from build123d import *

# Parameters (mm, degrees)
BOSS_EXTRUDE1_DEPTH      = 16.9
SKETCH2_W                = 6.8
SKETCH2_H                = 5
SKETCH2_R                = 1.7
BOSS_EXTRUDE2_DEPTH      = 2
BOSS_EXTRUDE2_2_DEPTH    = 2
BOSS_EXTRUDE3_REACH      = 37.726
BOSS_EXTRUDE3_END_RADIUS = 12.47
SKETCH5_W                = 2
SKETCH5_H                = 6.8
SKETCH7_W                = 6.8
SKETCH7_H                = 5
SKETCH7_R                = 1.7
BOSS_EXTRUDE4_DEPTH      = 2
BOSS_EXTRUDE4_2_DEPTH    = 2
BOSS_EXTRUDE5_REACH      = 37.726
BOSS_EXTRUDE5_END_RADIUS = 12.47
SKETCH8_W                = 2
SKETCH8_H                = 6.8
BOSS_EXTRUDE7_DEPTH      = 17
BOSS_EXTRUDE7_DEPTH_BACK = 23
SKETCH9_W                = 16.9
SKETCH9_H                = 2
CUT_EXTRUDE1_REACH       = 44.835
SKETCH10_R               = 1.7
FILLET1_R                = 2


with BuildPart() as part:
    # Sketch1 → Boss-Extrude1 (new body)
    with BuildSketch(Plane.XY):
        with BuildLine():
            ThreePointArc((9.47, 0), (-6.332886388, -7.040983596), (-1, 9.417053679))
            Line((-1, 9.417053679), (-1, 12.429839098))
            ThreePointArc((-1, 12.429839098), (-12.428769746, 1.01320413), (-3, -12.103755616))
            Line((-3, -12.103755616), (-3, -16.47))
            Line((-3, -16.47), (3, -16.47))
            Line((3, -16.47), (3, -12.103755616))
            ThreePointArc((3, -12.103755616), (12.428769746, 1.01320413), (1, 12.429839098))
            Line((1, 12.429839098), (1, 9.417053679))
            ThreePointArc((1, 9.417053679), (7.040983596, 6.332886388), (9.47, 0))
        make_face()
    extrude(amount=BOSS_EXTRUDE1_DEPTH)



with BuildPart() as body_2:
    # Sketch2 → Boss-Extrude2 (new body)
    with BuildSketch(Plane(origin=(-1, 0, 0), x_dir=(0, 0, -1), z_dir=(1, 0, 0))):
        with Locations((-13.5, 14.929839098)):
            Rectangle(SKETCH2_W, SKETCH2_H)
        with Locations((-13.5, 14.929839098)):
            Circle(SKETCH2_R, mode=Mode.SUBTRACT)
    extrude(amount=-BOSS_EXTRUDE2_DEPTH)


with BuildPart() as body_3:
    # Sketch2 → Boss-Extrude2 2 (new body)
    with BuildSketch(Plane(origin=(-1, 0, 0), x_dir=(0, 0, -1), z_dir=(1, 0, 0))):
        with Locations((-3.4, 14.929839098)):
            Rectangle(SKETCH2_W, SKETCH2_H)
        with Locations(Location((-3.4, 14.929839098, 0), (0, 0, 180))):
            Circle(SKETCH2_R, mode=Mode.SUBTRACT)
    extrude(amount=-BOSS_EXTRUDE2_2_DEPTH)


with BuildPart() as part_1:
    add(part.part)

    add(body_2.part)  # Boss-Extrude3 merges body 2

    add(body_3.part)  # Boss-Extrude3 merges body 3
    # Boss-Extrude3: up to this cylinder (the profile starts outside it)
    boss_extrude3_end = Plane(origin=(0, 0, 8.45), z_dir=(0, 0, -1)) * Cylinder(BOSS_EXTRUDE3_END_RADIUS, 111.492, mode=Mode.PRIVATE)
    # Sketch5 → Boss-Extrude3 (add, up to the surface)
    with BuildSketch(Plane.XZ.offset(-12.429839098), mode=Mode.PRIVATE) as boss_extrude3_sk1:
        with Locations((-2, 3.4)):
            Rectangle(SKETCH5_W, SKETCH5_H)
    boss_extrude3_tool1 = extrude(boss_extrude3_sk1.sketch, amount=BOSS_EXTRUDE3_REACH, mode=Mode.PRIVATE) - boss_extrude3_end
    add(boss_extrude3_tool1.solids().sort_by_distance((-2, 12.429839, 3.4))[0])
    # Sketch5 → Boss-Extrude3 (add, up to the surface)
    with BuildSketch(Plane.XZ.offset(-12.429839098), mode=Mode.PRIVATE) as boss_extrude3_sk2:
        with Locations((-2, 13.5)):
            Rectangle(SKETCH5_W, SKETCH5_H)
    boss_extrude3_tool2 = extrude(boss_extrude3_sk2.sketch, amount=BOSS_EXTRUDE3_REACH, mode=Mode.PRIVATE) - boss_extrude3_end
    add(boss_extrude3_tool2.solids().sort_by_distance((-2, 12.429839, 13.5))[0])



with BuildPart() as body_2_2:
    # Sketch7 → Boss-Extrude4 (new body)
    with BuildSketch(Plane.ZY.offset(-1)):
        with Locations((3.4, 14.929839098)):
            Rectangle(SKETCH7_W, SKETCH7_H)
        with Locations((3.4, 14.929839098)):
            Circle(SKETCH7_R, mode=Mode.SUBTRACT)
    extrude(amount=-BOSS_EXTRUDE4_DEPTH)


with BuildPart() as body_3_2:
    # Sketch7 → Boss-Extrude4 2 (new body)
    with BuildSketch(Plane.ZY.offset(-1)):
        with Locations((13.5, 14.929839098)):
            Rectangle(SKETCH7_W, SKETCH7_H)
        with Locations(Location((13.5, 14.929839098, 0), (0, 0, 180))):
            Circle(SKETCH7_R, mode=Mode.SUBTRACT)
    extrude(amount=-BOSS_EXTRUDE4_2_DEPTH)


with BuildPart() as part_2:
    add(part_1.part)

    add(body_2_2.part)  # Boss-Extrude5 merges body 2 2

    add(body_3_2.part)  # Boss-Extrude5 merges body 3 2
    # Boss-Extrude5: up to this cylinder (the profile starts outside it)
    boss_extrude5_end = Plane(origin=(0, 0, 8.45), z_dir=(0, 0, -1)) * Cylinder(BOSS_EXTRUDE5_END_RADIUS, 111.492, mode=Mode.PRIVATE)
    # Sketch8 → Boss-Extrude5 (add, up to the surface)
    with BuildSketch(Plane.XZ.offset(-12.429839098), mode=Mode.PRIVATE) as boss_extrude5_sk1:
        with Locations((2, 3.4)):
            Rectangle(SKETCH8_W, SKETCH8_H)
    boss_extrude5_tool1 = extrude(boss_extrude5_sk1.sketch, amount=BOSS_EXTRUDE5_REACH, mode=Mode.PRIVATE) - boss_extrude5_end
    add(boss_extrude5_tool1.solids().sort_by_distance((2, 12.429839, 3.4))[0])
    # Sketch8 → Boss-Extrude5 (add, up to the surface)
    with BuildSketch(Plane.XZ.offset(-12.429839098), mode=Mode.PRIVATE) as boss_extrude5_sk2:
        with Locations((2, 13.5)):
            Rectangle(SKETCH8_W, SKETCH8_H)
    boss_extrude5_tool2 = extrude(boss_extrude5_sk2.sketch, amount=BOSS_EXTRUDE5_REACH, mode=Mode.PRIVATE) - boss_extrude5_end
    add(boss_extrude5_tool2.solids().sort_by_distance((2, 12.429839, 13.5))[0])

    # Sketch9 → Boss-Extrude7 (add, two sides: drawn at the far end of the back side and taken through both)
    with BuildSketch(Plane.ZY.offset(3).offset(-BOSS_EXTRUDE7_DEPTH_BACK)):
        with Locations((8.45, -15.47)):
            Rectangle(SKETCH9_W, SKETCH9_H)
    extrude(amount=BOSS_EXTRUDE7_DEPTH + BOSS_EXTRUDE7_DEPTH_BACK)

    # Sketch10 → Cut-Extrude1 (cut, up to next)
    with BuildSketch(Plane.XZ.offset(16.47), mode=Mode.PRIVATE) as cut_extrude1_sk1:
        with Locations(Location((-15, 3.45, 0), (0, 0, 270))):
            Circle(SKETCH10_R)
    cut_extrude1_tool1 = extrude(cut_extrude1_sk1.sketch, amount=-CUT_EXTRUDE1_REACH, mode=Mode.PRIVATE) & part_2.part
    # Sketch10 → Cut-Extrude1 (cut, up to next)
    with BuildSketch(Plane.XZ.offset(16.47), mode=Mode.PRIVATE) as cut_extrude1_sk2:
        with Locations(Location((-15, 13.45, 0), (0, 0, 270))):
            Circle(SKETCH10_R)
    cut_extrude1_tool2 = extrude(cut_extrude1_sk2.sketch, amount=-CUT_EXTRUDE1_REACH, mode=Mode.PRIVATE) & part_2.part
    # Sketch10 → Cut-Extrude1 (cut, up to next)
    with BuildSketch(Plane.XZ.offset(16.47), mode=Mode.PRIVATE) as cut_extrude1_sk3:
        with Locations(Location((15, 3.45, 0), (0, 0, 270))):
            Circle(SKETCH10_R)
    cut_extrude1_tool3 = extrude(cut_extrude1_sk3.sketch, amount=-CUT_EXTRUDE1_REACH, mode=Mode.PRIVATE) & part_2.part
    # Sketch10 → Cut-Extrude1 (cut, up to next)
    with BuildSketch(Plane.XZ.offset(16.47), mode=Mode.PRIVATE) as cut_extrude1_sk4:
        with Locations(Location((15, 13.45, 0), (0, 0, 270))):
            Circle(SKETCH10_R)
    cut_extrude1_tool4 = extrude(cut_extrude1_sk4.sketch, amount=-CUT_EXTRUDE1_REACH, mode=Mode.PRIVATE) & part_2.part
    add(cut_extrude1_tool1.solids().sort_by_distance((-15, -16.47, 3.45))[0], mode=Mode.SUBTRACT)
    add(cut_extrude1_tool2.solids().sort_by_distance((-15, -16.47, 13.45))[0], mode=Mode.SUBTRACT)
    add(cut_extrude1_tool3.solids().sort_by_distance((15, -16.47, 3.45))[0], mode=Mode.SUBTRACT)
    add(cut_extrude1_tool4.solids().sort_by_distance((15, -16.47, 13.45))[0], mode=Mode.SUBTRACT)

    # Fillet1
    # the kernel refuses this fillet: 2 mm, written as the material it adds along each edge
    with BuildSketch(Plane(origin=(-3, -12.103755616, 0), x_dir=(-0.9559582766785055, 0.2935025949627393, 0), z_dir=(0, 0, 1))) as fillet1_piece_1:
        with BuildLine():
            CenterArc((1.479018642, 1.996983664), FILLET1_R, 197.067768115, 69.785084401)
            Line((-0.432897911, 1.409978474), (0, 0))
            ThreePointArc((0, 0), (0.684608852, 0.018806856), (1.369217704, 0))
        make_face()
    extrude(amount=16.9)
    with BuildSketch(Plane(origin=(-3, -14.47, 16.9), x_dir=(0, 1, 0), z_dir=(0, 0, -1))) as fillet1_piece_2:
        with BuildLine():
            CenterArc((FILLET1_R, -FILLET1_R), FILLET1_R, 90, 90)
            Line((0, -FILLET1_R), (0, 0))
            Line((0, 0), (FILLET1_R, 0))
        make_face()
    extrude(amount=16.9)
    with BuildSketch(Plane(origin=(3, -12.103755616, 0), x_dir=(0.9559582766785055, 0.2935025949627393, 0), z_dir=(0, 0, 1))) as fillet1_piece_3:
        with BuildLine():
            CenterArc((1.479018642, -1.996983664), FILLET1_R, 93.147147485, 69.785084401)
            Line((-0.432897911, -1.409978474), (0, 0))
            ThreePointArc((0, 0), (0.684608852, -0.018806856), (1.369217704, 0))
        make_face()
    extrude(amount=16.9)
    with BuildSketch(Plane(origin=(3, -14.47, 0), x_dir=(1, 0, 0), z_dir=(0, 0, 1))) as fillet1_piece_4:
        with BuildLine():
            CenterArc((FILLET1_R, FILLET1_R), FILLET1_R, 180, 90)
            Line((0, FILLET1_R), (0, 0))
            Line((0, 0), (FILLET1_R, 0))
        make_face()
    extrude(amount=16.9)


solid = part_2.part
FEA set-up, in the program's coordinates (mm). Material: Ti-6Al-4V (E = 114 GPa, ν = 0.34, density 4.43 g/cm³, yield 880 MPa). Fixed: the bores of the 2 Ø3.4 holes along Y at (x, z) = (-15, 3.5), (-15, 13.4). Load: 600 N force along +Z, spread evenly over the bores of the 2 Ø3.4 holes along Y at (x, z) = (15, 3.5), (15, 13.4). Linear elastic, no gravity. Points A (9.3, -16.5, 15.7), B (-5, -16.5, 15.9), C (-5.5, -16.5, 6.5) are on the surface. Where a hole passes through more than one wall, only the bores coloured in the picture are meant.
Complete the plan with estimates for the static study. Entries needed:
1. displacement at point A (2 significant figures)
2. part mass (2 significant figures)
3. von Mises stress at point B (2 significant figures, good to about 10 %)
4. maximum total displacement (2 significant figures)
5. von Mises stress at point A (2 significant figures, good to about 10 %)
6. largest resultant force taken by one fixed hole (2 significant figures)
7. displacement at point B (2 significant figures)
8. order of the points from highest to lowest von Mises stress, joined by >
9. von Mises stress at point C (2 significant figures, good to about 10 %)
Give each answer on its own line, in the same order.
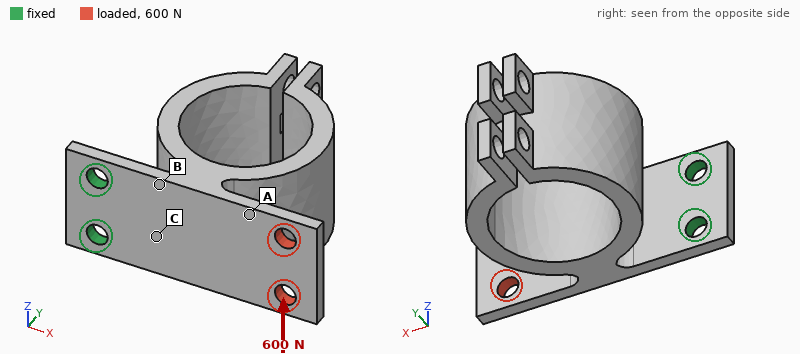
54 µm
23 g
95 MPa
86 µm
30 MPa
1.5 kN
18 µm
B > C > A
66 MPa
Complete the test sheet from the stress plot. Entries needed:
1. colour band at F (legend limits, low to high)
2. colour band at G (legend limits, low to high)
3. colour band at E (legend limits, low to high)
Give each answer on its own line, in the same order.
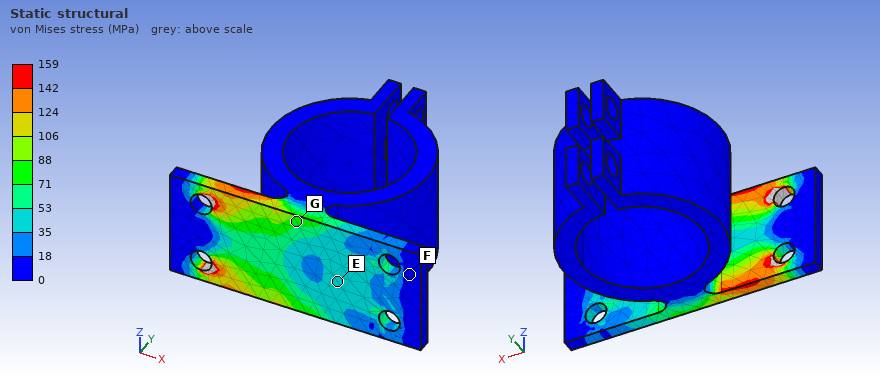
0 to 18 MPa
71 to 88 MPa
35 to 53 MPa
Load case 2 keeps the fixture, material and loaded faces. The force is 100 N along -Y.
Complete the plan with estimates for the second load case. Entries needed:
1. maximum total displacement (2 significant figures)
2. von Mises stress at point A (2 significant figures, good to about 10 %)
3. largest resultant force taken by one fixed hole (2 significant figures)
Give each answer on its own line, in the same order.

0.65 mm
52 MPa
51 N
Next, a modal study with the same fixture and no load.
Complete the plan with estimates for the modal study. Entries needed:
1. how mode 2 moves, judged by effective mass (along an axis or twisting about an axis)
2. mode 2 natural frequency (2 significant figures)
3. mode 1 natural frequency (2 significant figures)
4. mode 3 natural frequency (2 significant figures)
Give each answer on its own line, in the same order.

along Z
1300 Hz
600 Hz
2600 Hz
